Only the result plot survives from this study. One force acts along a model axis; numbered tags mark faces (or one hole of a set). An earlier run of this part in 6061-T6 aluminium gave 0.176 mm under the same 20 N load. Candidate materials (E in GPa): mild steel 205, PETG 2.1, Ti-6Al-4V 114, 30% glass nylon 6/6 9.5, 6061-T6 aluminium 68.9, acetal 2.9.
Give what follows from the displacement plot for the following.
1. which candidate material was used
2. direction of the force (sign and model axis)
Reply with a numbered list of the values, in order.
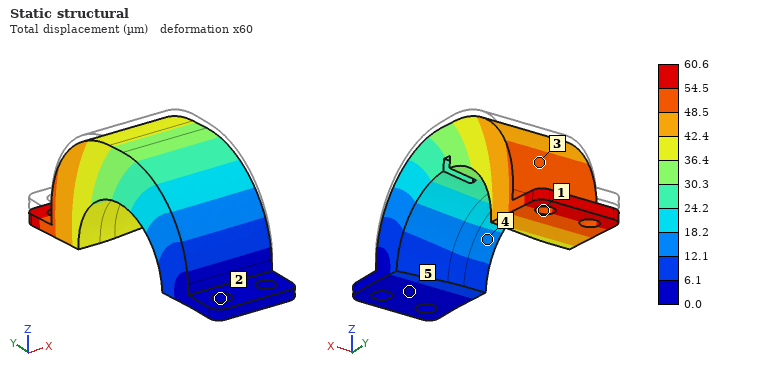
1. mild steel
2. -Z
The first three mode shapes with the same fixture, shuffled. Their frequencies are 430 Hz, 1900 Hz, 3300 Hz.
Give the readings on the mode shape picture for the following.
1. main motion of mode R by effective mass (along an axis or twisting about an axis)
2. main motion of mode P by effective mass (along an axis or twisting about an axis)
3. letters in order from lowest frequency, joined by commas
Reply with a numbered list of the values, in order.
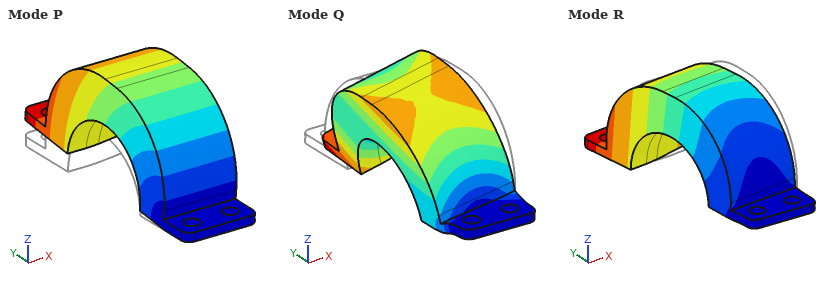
1. along X
2. along Z
3. P, R, Q
